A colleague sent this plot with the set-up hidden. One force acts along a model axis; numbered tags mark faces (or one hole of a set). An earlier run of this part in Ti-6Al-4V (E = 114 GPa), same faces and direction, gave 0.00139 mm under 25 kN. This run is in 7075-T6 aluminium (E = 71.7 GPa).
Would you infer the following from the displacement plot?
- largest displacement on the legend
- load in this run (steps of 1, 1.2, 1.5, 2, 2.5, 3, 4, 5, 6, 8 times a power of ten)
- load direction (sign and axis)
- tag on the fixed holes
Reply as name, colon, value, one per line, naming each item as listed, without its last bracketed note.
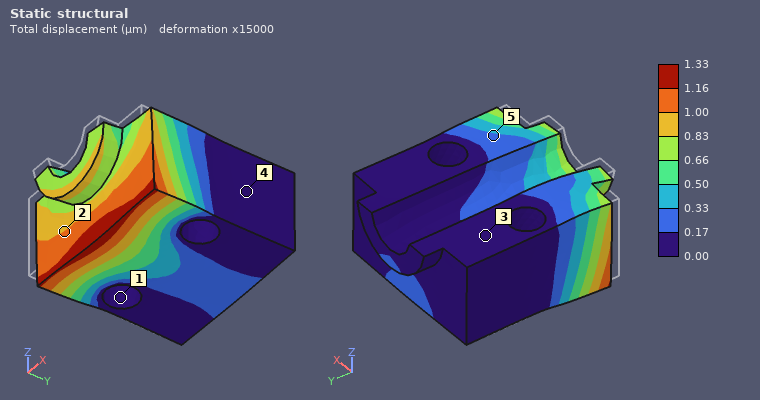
largest displacement on the legend: 1.33 µm
load in this run: 15 kN
load direction: +Y
tag on the fixed holes: 1
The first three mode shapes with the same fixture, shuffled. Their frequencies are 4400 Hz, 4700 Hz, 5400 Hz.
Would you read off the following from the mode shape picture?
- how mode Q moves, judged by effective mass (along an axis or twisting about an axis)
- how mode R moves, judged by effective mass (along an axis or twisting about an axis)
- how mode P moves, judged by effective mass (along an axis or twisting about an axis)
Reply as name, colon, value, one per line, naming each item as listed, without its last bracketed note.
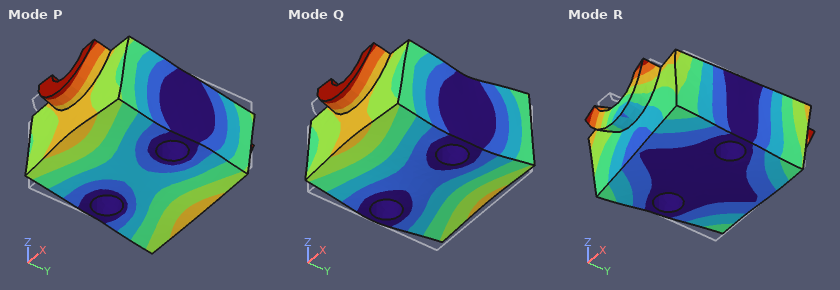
how mode Q moves, judged by effective mass: along Z
how mode R moves, judged by effective mass: twisting about Z
how mode P moves, judged by effective mass: twisting about X
